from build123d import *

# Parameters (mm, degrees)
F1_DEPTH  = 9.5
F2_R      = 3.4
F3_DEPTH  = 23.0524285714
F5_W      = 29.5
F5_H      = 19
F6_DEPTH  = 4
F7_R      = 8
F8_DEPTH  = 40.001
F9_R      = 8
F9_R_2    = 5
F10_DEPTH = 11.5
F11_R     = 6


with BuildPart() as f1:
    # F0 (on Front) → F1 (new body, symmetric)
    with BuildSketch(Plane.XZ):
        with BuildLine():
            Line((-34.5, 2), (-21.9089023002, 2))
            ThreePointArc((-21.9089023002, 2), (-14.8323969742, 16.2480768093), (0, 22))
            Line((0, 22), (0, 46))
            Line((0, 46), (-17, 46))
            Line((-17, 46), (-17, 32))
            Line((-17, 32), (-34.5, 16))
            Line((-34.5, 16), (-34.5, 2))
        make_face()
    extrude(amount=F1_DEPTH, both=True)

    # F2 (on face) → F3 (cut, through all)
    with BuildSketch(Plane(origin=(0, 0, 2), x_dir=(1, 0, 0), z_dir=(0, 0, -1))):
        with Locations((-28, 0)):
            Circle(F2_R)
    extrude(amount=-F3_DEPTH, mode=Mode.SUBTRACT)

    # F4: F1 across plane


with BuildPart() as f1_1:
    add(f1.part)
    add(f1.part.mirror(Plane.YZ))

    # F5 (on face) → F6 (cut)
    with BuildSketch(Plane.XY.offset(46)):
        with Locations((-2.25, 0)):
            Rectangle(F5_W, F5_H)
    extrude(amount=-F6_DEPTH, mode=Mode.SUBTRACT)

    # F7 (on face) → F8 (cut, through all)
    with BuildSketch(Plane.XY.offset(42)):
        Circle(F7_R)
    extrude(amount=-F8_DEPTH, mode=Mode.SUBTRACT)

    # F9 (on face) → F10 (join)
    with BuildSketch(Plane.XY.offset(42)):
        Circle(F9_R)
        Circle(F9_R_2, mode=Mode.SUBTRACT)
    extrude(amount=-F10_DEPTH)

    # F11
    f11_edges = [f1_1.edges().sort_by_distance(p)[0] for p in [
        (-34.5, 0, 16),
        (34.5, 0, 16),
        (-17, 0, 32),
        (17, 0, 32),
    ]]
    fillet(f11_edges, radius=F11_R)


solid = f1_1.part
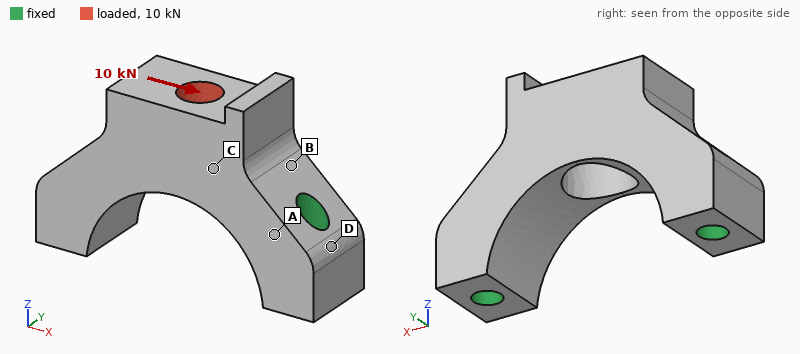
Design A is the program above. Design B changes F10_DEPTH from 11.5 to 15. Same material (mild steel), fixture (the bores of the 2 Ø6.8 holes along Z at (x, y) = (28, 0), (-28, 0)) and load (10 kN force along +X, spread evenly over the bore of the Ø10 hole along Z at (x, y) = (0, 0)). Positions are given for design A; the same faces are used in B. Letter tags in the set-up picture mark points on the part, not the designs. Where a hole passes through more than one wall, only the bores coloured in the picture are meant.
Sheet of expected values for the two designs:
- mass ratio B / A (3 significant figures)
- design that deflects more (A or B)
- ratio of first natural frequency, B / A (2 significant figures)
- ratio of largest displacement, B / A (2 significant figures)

1.02
A
0.99
0.82
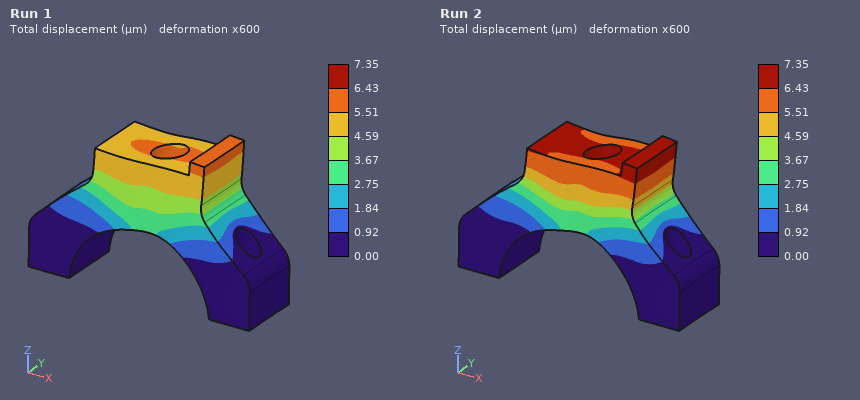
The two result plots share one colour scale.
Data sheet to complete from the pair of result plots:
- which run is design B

Run 1
